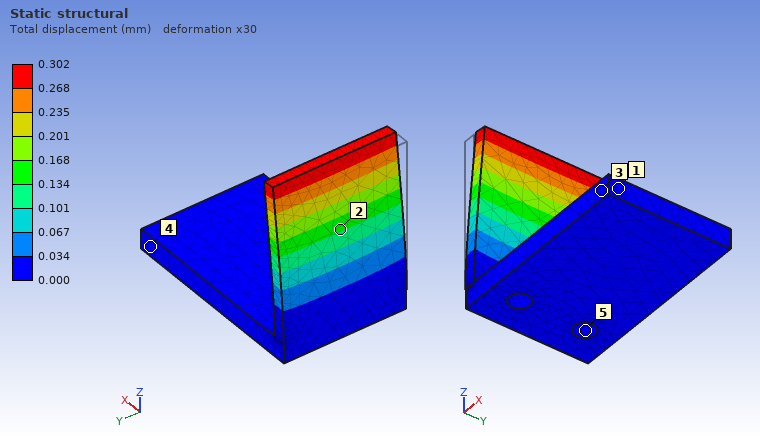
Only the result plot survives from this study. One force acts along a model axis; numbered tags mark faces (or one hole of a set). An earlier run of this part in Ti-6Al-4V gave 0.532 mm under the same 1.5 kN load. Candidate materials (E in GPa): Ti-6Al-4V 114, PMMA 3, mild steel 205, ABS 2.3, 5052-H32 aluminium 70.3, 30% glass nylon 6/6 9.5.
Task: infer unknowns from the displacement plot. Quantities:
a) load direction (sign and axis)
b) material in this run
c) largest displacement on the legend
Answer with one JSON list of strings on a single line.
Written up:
["+X", "mild steel", "0.302 mm"]
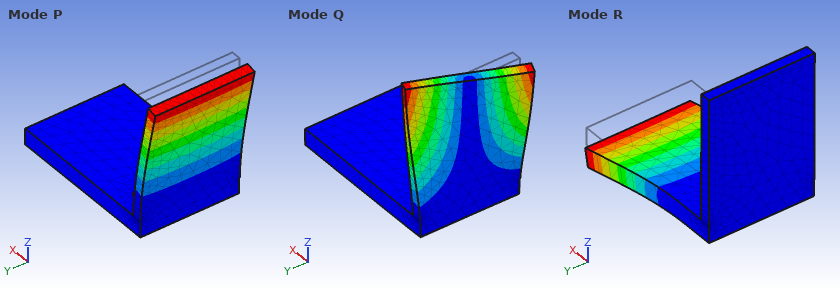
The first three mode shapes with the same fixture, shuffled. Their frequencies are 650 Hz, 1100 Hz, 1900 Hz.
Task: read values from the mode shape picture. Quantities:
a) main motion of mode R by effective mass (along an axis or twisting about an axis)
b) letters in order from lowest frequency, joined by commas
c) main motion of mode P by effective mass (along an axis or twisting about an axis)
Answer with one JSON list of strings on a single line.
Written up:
["along Z", "P, R, Q", "along X"]
